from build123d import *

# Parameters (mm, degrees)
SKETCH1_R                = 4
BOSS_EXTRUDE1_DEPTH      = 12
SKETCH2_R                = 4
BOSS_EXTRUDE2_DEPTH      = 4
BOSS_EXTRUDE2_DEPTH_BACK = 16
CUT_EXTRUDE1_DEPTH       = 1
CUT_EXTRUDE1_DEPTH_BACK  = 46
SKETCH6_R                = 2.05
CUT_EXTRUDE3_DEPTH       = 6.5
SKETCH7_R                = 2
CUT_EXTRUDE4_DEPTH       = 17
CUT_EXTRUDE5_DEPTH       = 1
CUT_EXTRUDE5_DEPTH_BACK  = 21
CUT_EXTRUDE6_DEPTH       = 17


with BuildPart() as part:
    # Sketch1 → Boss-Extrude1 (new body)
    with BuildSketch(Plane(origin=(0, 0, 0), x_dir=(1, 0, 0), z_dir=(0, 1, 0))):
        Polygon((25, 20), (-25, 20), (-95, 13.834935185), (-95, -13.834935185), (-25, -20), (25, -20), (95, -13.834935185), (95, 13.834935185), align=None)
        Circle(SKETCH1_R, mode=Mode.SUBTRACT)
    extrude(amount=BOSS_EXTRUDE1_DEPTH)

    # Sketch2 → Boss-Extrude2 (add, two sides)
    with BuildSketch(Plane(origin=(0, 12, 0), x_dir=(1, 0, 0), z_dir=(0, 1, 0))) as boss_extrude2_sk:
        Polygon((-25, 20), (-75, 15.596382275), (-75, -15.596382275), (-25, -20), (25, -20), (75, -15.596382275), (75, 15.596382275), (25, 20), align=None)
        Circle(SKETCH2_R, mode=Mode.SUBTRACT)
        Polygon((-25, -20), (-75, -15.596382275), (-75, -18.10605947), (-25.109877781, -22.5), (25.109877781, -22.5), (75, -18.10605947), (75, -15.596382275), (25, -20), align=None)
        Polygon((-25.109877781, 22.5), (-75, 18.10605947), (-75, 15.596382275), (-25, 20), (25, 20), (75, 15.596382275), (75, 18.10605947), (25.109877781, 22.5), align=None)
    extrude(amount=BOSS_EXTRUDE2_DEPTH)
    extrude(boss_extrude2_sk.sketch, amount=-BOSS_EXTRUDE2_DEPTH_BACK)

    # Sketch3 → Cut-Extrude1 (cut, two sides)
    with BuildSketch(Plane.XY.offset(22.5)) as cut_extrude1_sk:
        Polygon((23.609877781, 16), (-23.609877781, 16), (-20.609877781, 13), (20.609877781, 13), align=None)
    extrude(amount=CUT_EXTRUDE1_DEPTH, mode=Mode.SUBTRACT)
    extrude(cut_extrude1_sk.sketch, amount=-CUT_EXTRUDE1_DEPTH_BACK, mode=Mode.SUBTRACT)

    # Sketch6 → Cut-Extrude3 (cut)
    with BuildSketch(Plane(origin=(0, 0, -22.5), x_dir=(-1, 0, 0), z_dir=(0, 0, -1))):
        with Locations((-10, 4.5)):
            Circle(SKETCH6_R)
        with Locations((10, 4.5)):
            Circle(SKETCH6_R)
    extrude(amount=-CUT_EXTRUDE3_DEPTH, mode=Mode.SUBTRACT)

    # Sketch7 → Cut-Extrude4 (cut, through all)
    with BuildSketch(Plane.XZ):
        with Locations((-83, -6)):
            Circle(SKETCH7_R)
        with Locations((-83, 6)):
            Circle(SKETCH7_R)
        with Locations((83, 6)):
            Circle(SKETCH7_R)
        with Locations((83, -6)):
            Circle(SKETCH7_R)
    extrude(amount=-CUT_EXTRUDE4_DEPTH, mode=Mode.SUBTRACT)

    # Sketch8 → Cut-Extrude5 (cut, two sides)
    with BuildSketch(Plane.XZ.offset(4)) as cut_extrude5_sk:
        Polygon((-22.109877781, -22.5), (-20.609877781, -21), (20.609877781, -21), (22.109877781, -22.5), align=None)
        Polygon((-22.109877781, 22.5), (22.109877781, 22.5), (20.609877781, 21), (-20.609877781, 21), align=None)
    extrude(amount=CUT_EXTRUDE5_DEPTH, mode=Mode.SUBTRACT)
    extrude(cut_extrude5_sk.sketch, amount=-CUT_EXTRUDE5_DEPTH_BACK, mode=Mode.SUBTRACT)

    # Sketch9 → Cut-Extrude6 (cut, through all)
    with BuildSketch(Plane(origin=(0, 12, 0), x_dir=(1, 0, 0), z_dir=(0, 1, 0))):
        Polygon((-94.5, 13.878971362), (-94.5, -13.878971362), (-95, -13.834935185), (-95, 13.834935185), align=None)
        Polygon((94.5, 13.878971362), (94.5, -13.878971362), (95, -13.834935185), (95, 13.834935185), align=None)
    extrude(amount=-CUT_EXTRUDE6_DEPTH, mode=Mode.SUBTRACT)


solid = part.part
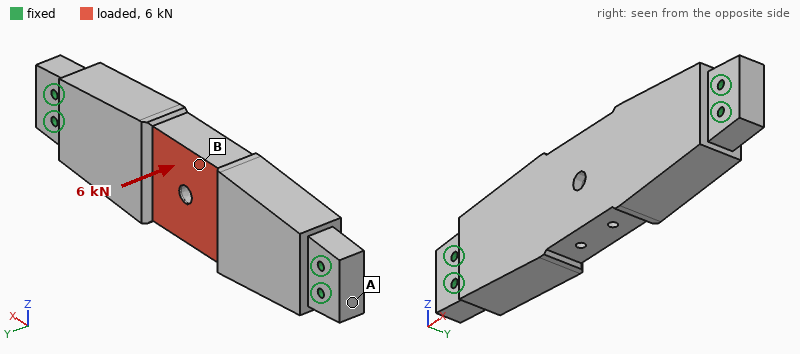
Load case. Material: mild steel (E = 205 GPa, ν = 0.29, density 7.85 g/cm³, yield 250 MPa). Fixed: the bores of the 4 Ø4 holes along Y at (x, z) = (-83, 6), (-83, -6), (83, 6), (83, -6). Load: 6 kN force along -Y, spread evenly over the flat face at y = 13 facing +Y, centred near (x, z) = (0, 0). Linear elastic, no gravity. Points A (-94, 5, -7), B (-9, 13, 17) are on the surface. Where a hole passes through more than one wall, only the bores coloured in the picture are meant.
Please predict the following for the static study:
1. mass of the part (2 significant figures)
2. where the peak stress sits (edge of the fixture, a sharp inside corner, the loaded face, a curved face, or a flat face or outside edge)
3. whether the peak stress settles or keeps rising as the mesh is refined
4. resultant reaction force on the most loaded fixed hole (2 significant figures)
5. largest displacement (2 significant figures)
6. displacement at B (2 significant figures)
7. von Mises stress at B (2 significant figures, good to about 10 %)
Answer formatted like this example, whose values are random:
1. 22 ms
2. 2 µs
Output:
1. 1.0 kg
2. edge of the fixture
3. keeps rising
4. 1.8 kN
5. 69 µm
6. 67 µm
7. 60 MPa
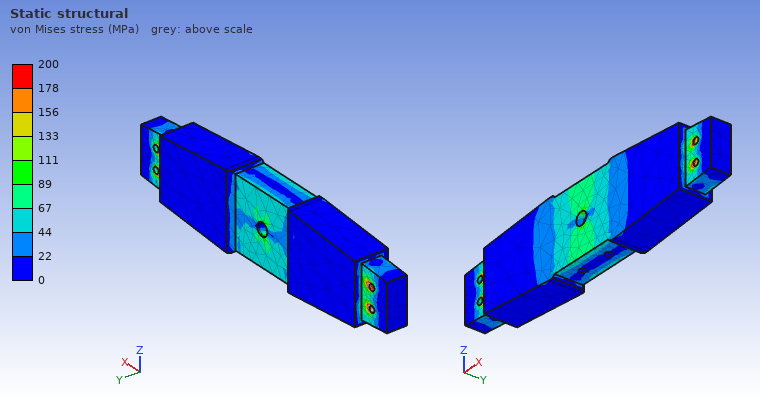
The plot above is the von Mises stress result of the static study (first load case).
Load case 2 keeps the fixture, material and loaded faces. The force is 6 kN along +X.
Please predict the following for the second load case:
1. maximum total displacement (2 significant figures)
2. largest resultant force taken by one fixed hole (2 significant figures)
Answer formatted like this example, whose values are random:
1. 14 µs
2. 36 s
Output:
1. 2.5 µm
2. 1.5 kN
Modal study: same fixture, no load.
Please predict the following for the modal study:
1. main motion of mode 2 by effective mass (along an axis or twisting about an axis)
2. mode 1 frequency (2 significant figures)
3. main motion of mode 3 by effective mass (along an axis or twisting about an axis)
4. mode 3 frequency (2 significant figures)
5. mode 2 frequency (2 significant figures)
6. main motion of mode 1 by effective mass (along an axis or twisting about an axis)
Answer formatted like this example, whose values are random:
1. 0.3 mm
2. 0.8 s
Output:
1. along Z
2. 2200 Hz
3. twisting about X
4. 5300 Hz
5. 4200 Hz
6. along Y
